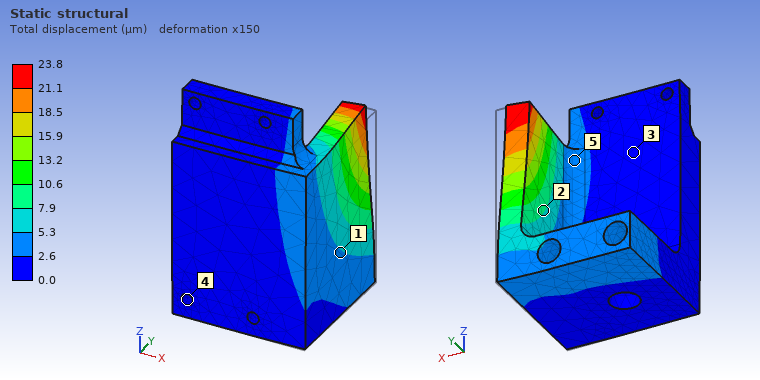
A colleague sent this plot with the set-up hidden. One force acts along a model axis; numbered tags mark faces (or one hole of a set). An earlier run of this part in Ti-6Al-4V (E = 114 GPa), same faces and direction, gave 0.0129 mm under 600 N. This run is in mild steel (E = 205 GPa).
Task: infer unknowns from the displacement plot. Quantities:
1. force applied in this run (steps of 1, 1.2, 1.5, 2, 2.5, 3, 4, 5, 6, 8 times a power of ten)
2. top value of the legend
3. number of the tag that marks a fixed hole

2 kN
23.8 µm
4
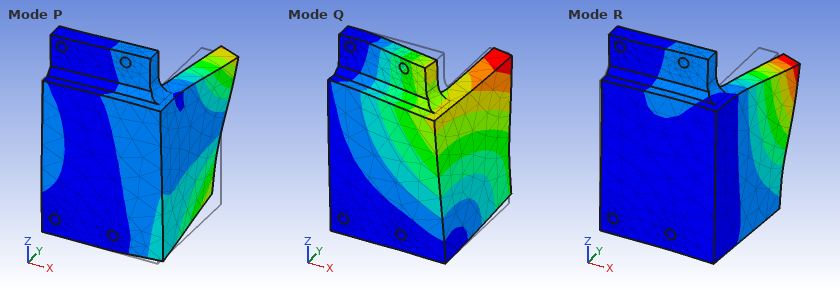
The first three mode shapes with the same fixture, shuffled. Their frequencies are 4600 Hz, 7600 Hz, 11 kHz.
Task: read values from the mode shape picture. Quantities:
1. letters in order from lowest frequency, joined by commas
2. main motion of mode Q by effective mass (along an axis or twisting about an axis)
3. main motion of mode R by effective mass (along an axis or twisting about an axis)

Q, R, P
along Y
along X
